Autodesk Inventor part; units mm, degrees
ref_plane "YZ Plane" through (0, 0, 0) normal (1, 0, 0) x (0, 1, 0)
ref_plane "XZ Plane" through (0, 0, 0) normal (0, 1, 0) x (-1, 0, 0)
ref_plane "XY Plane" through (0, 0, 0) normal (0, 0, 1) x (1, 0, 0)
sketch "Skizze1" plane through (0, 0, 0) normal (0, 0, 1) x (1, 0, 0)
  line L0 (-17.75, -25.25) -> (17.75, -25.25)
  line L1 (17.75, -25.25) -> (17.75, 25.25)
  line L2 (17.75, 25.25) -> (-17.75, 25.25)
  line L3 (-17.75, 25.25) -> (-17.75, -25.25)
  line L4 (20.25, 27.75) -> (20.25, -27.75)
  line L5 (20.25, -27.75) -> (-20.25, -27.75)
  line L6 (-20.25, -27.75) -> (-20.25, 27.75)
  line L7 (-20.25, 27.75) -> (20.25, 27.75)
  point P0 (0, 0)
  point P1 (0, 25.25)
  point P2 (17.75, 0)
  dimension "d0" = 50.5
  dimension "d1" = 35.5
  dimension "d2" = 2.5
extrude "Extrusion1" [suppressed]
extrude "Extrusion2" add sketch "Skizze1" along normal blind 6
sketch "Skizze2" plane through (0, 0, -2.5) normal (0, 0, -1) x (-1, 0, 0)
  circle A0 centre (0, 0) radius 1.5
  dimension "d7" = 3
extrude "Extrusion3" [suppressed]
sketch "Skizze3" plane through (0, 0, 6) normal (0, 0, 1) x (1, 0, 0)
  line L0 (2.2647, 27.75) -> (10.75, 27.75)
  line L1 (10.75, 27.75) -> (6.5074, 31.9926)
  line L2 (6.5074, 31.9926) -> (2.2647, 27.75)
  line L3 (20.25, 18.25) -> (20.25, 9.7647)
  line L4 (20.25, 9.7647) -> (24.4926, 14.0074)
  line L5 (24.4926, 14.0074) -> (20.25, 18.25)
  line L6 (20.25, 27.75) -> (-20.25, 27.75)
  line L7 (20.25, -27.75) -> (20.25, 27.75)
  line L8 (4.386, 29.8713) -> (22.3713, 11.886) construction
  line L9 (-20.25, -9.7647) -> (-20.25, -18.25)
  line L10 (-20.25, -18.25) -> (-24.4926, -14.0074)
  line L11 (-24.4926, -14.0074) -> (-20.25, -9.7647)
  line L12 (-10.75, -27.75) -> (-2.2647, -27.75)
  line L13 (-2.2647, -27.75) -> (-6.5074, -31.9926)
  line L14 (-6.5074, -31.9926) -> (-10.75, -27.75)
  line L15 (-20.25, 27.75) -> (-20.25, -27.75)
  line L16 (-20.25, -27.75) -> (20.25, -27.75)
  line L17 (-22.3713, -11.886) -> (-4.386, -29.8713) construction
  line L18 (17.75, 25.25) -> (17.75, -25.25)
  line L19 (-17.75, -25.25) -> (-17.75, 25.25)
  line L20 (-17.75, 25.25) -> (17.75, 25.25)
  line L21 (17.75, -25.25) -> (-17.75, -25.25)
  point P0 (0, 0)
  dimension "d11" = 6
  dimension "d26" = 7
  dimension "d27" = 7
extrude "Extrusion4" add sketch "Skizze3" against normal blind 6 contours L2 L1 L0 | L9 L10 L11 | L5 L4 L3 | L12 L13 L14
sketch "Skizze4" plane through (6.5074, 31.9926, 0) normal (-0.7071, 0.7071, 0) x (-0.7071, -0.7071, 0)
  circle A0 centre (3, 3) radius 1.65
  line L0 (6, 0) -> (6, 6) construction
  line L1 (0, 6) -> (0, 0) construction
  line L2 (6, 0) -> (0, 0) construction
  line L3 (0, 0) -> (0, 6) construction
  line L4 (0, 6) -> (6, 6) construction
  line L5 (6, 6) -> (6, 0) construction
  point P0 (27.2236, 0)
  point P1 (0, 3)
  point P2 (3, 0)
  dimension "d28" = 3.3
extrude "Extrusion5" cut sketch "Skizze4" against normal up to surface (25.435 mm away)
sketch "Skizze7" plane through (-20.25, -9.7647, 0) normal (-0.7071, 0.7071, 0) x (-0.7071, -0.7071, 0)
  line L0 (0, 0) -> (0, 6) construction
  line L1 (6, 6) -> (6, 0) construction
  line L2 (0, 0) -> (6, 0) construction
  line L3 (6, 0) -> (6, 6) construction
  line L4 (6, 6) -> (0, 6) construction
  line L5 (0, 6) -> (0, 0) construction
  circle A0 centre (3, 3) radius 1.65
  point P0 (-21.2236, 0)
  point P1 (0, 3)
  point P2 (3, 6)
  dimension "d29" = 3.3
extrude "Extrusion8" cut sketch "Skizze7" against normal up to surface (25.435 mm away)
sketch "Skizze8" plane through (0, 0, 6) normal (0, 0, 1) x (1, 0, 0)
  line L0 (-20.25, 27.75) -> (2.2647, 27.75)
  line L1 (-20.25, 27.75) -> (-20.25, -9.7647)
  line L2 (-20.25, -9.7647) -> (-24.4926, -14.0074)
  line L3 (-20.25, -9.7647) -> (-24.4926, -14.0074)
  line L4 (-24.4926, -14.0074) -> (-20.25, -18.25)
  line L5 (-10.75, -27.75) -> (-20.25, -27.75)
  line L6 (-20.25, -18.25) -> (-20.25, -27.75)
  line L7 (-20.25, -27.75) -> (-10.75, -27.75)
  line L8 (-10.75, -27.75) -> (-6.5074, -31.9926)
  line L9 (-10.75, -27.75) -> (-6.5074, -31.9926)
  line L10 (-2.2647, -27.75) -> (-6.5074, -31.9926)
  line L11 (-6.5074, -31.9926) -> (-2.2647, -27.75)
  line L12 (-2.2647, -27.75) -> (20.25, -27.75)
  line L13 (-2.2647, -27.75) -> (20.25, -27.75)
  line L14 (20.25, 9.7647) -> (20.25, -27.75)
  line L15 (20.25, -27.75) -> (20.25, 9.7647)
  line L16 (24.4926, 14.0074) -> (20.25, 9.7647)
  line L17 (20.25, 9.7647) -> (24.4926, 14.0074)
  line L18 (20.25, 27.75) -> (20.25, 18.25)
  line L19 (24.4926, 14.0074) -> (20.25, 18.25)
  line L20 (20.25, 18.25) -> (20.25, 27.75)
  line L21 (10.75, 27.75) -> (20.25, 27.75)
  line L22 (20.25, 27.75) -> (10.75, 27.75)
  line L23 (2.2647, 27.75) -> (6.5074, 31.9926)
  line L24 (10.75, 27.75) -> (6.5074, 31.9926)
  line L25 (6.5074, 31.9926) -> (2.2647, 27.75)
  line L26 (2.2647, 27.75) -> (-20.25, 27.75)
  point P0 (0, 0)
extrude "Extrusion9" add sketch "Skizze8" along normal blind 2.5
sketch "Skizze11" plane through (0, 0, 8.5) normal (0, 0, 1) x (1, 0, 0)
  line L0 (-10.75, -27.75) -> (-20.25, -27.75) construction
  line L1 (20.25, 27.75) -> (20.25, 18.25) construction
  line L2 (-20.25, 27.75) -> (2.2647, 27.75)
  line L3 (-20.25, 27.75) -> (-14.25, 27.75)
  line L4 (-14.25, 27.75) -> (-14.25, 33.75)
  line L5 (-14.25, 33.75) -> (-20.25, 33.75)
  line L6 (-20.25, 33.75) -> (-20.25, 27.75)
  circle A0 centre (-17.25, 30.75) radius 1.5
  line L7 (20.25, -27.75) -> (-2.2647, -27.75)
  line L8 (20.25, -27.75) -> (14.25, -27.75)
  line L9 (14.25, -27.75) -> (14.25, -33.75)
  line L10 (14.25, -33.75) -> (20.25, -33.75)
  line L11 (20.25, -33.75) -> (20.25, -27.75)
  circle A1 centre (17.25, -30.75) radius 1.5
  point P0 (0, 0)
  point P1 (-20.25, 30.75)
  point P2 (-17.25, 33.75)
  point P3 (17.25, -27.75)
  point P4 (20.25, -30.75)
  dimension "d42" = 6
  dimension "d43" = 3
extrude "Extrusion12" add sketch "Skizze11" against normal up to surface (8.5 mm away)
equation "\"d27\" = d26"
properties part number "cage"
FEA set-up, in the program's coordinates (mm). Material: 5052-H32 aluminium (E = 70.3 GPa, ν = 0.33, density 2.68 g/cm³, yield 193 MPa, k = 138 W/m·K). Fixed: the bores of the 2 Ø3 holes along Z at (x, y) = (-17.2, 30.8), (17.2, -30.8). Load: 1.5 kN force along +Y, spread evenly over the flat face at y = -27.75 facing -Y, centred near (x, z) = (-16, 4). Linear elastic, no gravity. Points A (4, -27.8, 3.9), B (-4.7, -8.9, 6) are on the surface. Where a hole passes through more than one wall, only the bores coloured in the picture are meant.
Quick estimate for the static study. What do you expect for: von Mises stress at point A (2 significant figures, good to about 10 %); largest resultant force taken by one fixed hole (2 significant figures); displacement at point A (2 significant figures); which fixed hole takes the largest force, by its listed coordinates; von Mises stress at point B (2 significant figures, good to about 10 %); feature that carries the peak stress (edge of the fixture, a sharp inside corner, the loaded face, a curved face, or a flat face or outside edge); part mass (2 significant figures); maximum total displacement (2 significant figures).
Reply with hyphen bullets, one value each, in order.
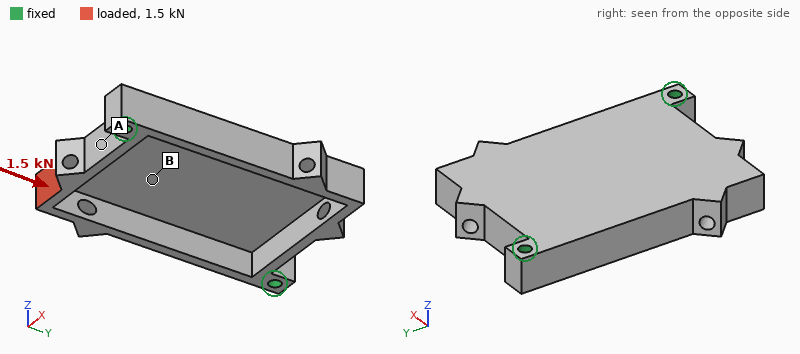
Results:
- 36 MPa
- 1.1 kN
- 21 µm
- (-17.2, 30.8)
- 17 MPa
- a curved face
- 25 g
- 79 µm
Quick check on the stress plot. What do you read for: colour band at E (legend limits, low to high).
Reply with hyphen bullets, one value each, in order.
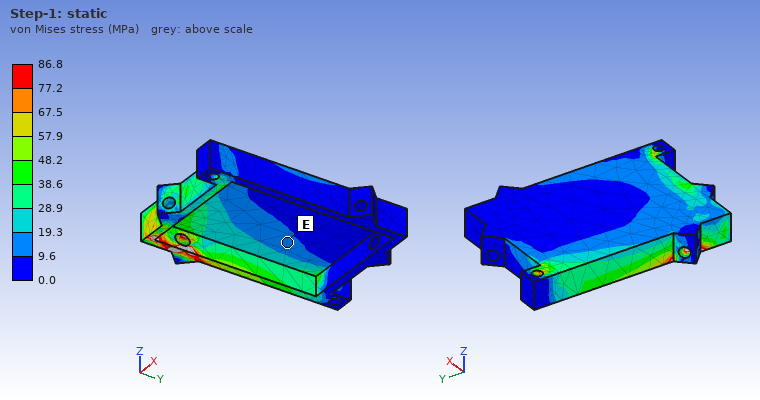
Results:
- 9.6 to 19.3 MPa
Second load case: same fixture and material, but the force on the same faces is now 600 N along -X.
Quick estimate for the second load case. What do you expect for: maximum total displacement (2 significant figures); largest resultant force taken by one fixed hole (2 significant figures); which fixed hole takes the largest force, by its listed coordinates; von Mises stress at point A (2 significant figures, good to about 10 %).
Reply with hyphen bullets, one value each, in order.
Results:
- 25 µm
- 560 N
- (17.2, -30.8)
- 23 MPa
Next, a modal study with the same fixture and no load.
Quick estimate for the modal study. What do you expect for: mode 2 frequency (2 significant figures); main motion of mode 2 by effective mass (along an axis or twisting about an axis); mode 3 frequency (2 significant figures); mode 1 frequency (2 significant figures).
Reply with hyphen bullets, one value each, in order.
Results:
- 3600 Hz
- along Z
- 7300 Hz
- 3100 Hz
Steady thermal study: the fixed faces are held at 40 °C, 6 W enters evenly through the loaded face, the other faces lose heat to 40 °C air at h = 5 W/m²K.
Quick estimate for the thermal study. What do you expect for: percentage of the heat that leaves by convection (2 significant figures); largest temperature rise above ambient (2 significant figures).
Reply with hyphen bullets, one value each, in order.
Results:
- 4.2 %
- 20 K
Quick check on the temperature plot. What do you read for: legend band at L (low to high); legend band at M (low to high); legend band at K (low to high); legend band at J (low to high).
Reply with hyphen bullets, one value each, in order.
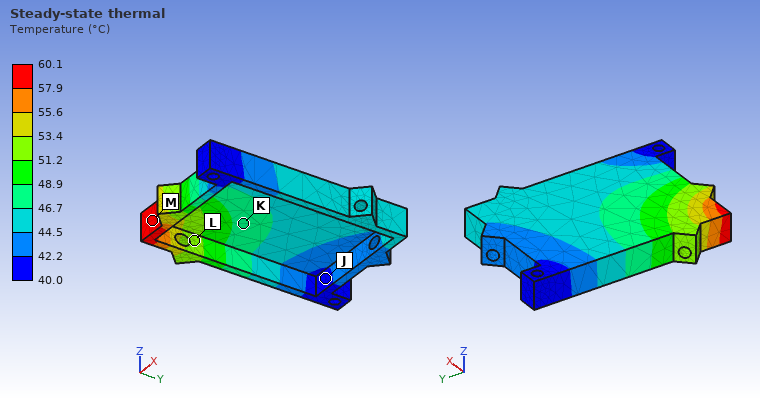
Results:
- 51.2 to 53.4 °C
- 57.9 to 60.1 °C
- 46.7 to 48.9 °C
- 40.0 to 42.2 °C
